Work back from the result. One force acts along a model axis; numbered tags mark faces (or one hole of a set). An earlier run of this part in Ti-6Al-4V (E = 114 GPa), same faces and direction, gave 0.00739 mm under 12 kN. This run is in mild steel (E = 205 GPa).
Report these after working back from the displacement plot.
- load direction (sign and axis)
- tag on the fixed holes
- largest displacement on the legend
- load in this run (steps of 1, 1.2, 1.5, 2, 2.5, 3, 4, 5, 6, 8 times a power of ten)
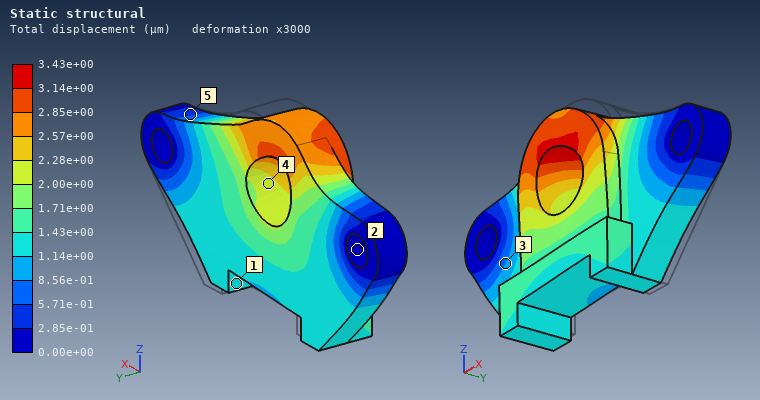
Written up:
-X
2
3.43e+00 µm
10 kN
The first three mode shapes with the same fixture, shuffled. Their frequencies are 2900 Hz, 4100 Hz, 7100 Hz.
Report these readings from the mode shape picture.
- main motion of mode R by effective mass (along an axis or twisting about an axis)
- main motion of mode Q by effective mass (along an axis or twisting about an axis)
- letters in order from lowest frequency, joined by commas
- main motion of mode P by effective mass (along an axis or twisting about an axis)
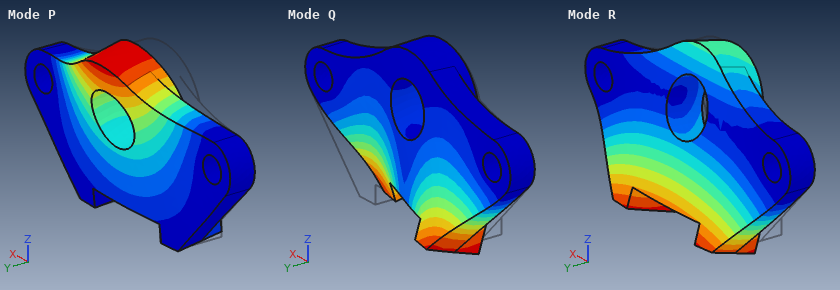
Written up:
along Y
twisting about Z
R, P, Q
along Y
